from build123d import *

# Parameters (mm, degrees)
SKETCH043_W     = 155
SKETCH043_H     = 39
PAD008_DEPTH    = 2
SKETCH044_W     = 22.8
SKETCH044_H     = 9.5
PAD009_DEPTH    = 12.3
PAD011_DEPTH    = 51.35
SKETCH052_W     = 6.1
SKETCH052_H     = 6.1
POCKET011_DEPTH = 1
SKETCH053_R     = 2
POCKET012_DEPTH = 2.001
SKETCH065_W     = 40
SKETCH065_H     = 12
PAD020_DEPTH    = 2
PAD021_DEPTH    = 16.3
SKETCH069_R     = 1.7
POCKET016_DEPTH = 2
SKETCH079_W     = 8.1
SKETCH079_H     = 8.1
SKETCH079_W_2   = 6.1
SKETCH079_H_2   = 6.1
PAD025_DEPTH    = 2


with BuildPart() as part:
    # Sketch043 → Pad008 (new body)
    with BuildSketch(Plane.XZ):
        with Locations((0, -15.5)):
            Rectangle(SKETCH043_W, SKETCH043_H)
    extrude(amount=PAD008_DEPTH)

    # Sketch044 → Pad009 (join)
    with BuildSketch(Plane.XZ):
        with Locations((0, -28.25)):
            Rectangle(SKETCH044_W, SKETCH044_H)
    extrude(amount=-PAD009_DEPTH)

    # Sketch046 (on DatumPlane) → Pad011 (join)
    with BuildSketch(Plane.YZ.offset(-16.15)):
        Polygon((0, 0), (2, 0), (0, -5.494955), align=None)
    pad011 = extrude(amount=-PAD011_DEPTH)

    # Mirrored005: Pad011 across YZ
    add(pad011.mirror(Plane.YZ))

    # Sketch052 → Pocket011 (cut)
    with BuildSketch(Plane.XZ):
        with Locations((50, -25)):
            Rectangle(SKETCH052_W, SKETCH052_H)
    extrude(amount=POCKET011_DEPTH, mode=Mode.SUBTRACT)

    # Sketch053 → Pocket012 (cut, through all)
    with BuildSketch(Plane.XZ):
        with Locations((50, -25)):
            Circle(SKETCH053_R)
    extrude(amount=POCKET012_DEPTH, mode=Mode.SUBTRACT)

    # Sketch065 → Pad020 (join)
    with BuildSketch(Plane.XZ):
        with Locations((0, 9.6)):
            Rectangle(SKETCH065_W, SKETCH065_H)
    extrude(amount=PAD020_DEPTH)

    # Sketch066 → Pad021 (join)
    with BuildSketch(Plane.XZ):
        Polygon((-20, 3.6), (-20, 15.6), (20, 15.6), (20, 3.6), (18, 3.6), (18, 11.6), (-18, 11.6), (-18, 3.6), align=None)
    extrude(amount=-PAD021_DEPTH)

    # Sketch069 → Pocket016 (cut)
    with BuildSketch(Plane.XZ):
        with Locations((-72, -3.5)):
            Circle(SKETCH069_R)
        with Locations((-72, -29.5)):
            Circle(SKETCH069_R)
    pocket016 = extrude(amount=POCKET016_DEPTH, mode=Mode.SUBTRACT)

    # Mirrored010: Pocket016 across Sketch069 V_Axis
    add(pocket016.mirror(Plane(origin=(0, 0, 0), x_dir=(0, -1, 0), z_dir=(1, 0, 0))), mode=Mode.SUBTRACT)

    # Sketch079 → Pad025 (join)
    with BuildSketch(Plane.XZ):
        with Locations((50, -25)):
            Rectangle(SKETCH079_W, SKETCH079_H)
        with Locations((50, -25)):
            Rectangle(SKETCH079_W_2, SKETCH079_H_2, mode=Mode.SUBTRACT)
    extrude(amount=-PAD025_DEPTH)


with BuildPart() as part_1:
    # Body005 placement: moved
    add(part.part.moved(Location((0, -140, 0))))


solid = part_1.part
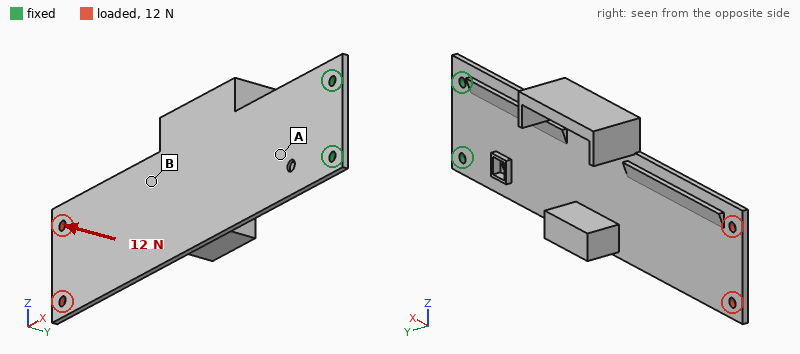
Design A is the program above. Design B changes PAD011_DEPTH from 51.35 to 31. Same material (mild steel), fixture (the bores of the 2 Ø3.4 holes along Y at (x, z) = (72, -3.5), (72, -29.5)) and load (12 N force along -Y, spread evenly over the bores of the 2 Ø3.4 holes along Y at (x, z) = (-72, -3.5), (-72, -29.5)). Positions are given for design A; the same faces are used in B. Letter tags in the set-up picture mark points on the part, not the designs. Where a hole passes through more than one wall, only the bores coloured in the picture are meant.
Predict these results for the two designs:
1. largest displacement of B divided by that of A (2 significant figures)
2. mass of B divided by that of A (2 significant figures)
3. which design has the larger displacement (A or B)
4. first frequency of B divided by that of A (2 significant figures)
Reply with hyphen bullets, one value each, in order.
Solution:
- 1.2
- 0.99
- B
- 0.92
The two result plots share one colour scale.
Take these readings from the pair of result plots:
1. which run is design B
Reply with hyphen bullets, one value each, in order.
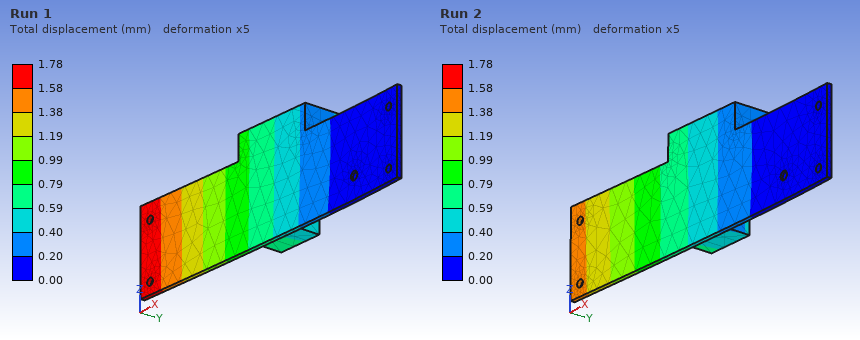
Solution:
- Run 1
